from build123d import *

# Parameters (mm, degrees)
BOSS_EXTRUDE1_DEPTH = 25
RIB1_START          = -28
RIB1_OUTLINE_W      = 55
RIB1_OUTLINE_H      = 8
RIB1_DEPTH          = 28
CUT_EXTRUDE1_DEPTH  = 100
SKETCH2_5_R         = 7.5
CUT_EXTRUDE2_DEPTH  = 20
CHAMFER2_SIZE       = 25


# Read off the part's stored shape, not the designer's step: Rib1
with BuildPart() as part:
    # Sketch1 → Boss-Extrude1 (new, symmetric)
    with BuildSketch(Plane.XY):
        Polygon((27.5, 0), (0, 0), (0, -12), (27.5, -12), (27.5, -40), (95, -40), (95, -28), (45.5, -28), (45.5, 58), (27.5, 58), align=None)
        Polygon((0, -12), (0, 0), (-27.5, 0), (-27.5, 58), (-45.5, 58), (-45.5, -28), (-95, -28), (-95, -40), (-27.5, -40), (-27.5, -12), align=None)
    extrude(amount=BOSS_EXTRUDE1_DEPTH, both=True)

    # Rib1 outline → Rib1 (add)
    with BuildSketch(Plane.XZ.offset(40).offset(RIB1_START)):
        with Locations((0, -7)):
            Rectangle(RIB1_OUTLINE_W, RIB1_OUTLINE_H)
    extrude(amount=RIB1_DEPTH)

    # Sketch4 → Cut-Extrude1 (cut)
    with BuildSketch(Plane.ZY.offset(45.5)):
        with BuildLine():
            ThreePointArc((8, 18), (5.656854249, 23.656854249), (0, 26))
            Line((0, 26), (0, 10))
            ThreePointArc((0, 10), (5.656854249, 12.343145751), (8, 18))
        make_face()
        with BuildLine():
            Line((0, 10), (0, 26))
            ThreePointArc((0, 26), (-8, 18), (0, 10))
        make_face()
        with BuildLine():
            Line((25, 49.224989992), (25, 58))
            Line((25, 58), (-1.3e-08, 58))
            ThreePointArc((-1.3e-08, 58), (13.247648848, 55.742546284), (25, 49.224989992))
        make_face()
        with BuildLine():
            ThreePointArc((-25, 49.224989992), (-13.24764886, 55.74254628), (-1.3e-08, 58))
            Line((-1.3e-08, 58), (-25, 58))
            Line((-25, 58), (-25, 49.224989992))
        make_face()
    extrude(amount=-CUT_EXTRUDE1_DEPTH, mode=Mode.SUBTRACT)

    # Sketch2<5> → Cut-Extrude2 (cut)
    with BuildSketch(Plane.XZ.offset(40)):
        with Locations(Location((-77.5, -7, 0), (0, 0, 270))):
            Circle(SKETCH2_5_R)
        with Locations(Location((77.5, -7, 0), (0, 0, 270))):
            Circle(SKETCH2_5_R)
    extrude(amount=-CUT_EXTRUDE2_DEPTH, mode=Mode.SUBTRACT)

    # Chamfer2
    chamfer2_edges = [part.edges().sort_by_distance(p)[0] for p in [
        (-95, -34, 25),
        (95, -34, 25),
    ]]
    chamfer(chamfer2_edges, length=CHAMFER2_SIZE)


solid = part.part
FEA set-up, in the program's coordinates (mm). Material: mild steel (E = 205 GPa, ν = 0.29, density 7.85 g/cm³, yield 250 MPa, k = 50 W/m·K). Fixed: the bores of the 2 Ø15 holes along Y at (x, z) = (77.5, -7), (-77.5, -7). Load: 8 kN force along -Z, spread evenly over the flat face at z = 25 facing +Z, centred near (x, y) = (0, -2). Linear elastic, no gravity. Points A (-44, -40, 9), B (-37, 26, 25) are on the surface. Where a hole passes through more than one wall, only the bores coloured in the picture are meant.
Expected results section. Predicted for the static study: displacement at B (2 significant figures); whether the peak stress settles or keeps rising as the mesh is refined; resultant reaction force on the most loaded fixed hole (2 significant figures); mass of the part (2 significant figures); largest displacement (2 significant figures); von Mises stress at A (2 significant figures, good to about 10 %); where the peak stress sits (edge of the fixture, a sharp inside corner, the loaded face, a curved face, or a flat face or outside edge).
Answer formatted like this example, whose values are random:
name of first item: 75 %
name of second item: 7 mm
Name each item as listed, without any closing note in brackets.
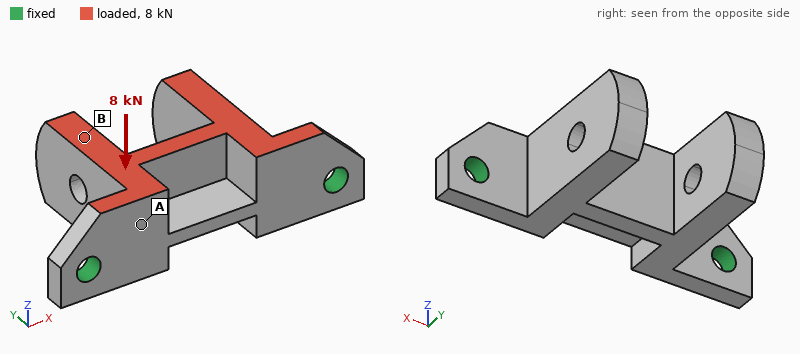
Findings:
displacement at B: 0.13 mm
whether the peak stress settles or keeps rising as the mesh is refined: keeps rising
resultant reaction force on the most loaded fixed hole: 4.0 kN
mass of the part: 2.0 kg
largest displacement: 0.18 mm
von Mises stress at A: 40 MPa
where the peak stress sits: edge of the fixture
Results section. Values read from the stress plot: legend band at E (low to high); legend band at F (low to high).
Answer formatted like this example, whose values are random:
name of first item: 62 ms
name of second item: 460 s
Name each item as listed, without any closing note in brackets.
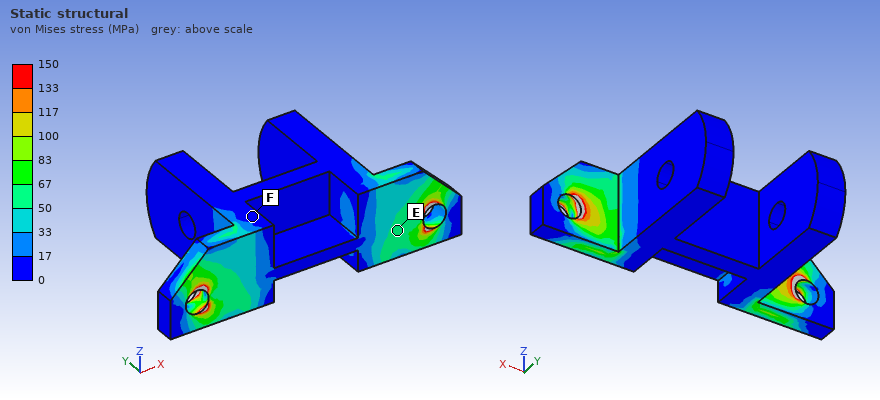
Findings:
legend band at E: 50 to 67 MPa
legend band at F: 0 to 17 MPa
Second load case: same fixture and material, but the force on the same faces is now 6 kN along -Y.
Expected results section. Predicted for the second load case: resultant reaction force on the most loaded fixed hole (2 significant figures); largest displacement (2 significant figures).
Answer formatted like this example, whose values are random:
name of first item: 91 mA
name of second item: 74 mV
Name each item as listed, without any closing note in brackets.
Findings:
resultant reaction force on the most loaded fixed hole: 3.6 kN
largest displacement: 0.11 mm
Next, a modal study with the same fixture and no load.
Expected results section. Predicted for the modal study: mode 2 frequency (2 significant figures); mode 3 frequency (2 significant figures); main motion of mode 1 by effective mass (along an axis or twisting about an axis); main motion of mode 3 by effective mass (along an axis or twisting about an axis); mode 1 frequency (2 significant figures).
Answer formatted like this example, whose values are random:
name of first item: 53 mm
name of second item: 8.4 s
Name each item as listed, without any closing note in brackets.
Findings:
mode 2 frequency: 1900 Hz
mode 3 frequency: 2200 Hz
main motion of mode 1 by effective mass: along Z
main motion of mode 3 by effective mass: along X
mode 1 frequency: 940 Hz
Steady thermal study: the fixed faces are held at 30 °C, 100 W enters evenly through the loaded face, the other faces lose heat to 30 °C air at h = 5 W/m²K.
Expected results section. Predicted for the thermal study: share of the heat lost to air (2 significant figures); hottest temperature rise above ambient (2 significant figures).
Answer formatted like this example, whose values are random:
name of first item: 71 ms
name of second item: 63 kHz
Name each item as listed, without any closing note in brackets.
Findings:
share of the heat lost to air: 12 %
hottest temperature rise above ambient: 87 K
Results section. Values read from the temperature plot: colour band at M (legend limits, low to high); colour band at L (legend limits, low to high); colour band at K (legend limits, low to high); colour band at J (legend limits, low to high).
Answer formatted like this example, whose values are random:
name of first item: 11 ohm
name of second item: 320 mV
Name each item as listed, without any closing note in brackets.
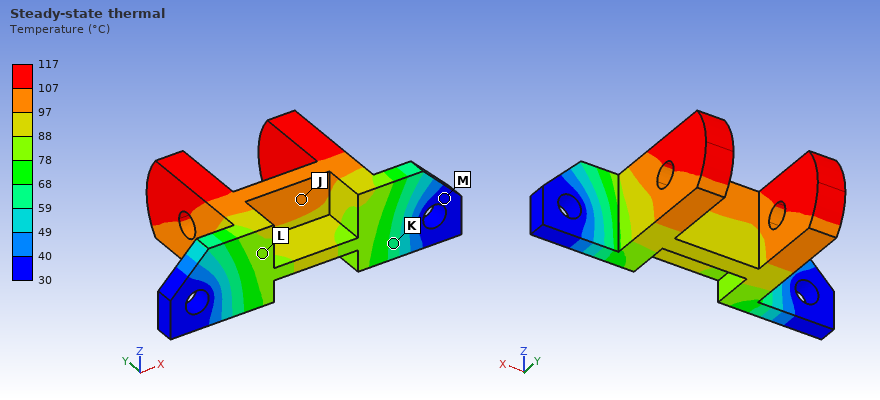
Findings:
colour band at M: 30 to 40 °C
colour band at L: 78 to 88 °C
colour band at K: 59 to 68 °C
colour band at J: 97 to 107 °C
